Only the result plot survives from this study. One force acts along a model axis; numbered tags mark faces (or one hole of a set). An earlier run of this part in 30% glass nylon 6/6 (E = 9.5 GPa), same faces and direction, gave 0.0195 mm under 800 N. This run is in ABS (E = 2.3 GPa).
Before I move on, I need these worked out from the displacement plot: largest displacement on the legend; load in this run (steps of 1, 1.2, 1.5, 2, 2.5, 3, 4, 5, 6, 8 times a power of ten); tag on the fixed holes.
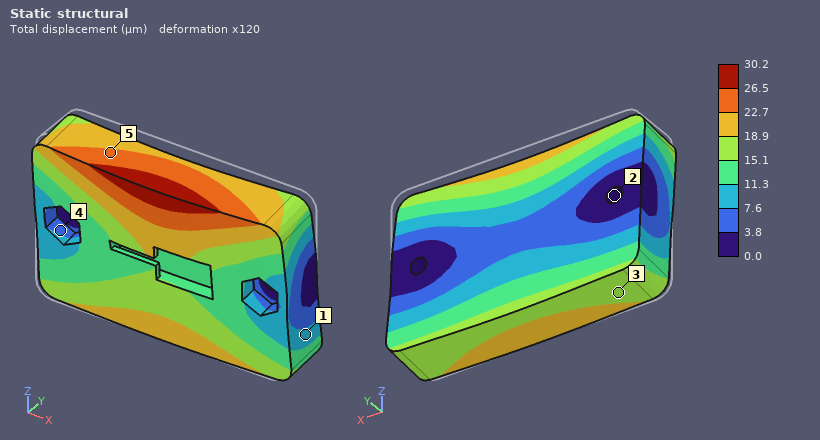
30.2 µm
300 N
2
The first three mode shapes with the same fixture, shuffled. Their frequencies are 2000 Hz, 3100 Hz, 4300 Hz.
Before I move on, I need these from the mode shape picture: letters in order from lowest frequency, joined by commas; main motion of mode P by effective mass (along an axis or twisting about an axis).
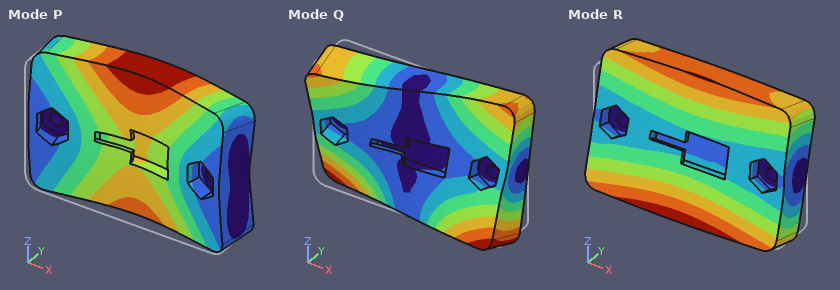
R, P, Q
along Y
